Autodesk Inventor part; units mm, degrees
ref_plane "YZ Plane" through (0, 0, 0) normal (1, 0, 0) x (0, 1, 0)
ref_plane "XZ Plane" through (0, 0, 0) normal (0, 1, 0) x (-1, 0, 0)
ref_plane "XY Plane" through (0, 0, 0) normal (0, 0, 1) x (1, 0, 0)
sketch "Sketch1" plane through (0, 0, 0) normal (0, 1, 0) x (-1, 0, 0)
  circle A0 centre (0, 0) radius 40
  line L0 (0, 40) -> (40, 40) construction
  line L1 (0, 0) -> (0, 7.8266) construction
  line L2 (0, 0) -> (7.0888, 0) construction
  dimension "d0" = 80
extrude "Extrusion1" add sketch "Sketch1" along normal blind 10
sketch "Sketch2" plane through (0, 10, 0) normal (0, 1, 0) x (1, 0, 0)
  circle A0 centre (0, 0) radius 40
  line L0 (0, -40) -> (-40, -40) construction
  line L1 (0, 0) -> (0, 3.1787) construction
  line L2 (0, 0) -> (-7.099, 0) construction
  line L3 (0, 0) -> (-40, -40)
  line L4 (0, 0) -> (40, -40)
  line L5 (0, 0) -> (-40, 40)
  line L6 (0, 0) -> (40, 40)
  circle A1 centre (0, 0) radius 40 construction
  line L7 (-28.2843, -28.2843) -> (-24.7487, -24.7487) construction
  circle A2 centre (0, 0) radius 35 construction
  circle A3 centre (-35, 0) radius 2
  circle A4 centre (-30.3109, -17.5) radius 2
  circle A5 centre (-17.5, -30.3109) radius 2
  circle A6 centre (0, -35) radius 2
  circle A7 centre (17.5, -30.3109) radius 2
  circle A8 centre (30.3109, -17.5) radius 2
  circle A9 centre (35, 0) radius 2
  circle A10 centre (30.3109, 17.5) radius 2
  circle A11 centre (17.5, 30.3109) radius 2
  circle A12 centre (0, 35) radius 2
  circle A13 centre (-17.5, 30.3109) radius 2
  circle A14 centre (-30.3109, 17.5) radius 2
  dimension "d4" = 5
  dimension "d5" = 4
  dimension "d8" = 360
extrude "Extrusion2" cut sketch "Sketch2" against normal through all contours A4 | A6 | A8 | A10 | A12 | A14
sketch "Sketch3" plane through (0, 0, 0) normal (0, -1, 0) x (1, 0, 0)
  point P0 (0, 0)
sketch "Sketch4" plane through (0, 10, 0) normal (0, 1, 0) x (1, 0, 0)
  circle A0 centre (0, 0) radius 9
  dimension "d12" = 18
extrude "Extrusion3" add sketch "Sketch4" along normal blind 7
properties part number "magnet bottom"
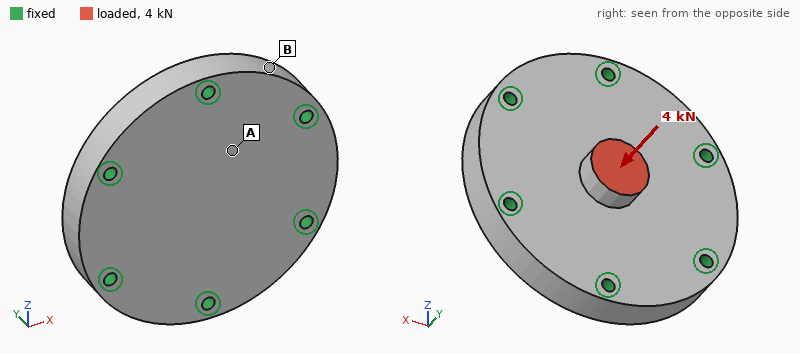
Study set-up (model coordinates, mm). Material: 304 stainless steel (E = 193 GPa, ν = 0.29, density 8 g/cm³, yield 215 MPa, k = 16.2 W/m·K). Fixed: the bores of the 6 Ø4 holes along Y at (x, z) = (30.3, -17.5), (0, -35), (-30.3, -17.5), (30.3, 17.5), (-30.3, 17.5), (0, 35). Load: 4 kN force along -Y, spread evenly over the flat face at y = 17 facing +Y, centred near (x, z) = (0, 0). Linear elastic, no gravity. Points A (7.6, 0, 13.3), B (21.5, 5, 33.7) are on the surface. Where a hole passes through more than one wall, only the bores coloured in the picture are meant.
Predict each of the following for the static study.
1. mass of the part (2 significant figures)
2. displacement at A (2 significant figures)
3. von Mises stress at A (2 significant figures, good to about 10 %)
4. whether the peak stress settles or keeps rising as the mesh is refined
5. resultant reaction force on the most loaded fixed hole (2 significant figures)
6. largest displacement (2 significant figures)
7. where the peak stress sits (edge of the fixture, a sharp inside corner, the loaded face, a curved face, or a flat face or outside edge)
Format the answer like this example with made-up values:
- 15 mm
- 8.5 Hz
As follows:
- 410 g
- 4.6 µm
- 16 MPa
- keeps rising
- 670 N
- 7.1 µm
- edge of the fixture
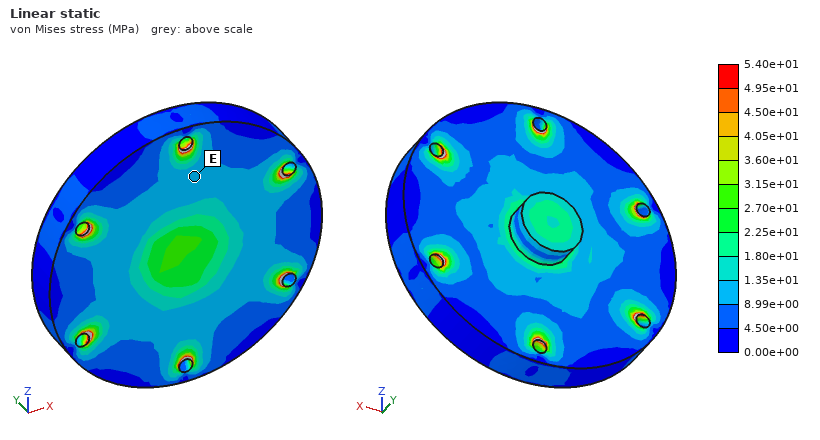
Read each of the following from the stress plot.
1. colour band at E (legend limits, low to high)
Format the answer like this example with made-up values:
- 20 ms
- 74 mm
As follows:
- 8.99e+00 to 1.35e+01 MPa
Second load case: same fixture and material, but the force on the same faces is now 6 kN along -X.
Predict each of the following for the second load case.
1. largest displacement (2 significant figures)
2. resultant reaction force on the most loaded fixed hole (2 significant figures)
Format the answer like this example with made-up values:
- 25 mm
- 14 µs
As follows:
- 11 µm
- 1.5 kN
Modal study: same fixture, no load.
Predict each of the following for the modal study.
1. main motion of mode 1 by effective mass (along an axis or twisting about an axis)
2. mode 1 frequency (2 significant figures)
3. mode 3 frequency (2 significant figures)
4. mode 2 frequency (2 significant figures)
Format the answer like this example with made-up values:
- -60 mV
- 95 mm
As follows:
- along Y
- 12 kHz
- 23 kHz
- 23 kHz
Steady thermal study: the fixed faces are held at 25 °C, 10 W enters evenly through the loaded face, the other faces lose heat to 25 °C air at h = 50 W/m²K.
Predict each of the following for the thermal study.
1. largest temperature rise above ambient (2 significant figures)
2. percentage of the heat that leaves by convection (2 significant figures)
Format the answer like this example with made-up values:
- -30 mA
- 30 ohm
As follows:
- 37 K
- 27 %
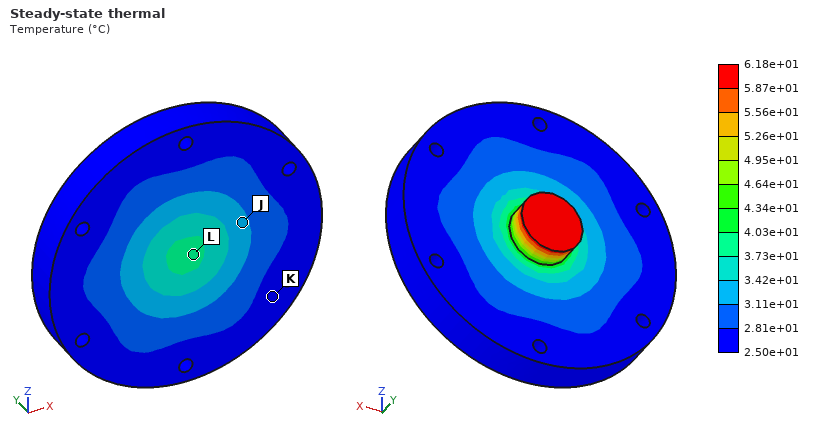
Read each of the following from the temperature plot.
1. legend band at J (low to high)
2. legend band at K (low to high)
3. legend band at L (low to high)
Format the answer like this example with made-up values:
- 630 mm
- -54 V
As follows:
- 3.11e+01 to 3.42e+01 °C
- 2.50e+01 to 2.81e+01 °C
- 3.73e+01 to 4.03e+01 °C
